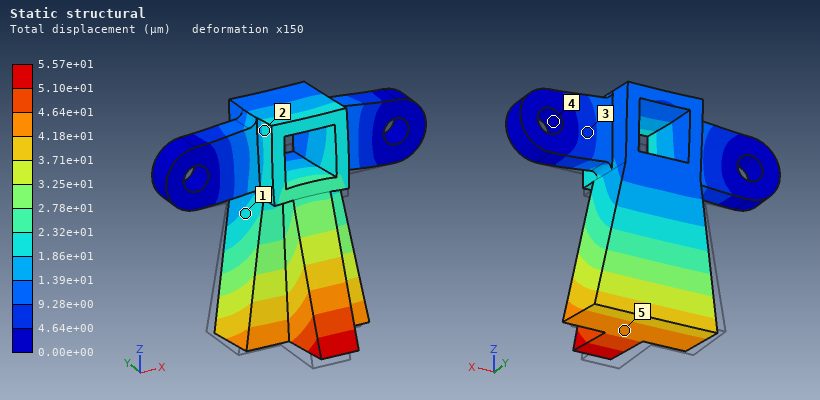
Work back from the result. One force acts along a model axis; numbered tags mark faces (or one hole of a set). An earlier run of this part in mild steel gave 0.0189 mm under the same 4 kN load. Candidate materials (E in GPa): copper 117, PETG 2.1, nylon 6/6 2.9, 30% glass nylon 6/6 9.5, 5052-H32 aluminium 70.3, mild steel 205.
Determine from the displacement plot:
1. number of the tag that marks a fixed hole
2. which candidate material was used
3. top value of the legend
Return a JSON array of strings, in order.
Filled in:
["4", "5052-H32 aluminium", "5.57e+01 µm"]
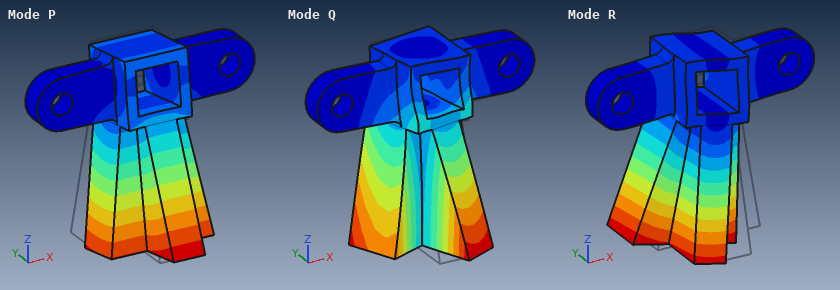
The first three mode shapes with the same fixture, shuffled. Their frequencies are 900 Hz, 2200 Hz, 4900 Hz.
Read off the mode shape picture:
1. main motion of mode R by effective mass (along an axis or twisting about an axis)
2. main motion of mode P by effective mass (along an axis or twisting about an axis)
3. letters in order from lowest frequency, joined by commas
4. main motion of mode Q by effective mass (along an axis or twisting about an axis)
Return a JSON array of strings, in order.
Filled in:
["along X", "along Y", "P, R, Q", "twisting about Z"]
